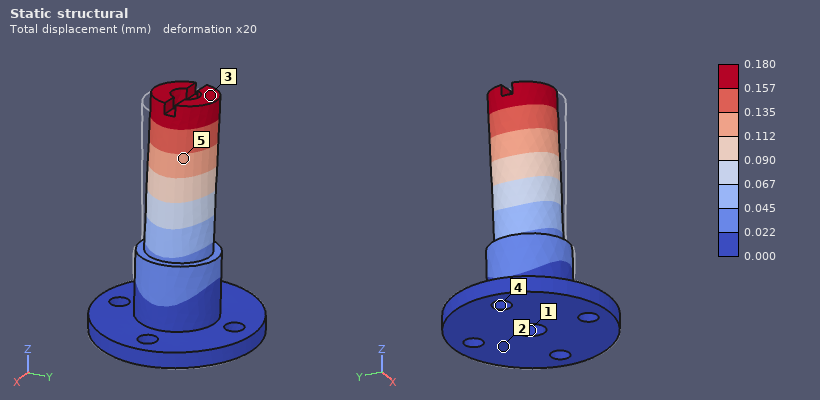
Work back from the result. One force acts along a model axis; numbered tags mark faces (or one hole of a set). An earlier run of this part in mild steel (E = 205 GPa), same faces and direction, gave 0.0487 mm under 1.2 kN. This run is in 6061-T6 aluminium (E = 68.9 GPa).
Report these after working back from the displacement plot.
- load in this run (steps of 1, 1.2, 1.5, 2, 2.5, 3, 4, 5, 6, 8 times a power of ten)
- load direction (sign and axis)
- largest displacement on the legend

1.5 kN
-X
0.180 mm
